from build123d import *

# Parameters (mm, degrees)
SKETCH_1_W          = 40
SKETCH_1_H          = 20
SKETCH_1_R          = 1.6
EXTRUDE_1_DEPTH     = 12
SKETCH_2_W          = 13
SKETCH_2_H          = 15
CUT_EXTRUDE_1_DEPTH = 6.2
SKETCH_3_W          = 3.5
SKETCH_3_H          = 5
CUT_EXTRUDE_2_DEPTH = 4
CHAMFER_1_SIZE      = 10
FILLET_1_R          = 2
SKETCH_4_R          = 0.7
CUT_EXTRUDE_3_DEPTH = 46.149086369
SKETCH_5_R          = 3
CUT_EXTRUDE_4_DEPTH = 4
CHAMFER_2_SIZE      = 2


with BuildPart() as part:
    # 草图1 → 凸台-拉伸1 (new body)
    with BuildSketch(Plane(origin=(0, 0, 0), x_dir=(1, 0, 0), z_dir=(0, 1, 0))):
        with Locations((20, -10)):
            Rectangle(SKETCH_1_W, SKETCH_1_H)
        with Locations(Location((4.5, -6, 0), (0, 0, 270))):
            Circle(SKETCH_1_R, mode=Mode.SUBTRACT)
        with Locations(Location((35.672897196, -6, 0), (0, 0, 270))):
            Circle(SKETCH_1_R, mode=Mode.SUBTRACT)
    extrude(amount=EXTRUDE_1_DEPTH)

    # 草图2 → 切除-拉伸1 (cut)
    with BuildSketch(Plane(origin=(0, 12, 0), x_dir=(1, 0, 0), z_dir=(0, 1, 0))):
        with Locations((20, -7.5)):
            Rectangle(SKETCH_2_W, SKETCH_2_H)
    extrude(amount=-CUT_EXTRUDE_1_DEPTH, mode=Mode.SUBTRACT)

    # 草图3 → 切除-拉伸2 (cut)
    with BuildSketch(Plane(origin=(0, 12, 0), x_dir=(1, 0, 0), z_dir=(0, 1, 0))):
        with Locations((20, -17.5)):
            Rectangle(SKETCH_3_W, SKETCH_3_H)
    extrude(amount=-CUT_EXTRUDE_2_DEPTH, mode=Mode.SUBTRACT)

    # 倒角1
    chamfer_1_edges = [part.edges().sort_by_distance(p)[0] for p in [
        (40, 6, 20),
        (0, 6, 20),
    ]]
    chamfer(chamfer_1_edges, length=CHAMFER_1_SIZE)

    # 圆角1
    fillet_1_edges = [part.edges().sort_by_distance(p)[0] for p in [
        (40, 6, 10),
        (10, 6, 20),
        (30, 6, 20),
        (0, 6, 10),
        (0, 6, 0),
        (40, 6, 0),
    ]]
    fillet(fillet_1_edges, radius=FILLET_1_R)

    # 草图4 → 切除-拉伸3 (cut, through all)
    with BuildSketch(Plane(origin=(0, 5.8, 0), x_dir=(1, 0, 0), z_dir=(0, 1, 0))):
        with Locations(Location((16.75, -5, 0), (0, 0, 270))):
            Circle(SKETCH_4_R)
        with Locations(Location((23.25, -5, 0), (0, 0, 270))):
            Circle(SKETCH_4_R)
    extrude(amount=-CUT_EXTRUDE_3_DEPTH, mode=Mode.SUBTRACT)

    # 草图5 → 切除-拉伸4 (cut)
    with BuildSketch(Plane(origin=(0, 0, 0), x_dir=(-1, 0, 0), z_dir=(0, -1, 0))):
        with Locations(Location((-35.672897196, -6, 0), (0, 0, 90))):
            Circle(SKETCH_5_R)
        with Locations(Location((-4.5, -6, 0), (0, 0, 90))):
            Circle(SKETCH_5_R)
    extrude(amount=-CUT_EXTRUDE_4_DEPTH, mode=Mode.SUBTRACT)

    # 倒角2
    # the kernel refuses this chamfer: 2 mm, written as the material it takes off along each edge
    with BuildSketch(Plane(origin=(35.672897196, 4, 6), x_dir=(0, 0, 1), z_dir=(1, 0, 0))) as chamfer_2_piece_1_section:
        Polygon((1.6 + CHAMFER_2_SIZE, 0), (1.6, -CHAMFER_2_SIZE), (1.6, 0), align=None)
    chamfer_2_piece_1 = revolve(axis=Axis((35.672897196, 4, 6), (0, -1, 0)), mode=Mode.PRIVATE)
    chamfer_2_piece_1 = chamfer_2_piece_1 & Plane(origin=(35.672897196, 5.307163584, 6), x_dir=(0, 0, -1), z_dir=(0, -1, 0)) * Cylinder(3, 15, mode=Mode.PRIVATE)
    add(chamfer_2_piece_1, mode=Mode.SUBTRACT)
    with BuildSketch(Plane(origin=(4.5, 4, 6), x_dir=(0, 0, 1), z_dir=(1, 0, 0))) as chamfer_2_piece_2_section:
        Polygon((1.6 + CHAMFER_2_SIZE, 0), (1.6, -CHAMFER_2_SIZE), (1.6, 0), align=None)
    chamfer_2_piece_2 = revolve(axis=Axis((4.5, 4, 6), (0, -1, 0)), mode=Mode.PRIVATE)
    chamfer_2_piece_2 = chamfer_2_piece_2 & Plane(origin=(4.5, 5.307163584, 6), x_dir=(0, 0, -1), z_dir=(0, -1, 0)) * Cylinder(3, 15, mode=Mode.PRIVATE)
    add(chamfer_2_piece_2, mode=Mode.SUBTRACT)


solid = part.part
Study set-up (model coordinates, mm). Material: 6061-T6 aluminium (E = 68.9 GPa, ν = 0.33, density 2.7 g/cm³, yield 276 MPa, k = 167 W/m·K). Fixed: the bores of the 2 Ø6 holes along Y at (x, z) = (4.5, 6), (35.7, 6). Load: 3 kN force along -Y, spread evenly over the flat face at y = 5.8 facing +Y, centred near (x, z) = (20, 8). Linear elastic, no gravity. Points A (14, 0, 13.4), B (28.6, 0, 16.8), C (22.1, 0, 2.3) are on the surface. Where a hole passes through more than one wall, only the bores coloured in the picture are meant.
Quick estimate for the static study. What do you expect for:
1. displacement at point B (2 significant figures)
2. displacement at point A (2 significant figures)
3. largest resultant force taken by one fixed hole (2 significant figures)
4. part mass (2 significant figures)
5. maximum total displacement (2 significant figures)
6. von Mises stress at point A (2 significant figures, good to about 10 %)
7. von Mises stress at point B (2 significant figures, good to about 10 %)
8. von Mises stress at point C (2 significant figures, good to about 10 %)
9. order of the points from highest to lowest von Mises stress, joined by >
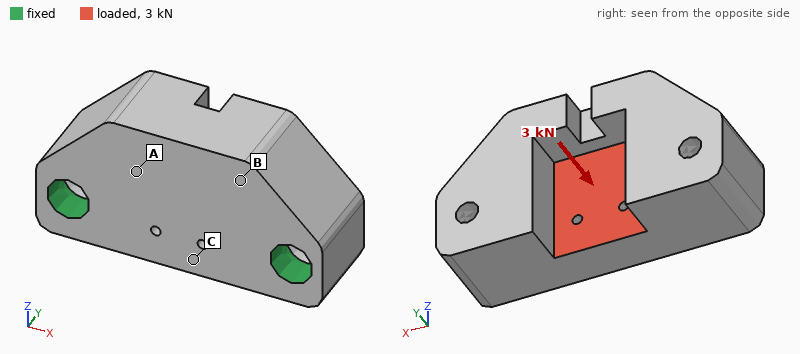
11 µm
13 µm
1.5 kN
18 g
19 µm
20 MPa
10 MPa
54 MPa
C > A > B
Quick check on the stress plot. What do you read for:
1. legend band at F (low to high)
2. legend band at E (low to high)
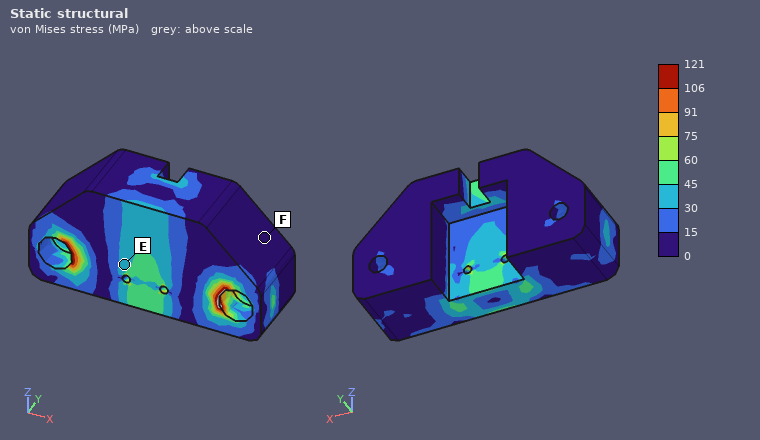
0 to 15 MPa
30 to 45 MPa
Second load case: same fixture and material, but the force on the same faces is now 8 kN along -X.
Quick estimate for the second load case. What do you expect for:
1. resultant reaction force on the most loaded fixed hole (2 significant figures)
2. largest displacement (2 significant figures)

4.1 kN
13 µm
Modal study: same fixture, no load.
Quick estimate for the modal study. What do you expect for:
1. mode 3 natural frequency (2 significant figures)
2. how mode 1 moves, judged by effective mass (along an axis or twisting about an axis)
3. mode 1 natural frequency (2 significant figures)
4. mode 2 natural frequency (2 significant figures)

33 kHz
along Y
19 kHz
31 kHz
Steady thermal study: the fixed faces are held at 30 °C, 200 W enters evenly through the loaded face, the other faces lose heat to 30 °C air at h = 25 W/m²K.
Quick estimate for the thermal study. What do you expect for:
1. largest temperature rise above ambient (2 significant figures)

72 K
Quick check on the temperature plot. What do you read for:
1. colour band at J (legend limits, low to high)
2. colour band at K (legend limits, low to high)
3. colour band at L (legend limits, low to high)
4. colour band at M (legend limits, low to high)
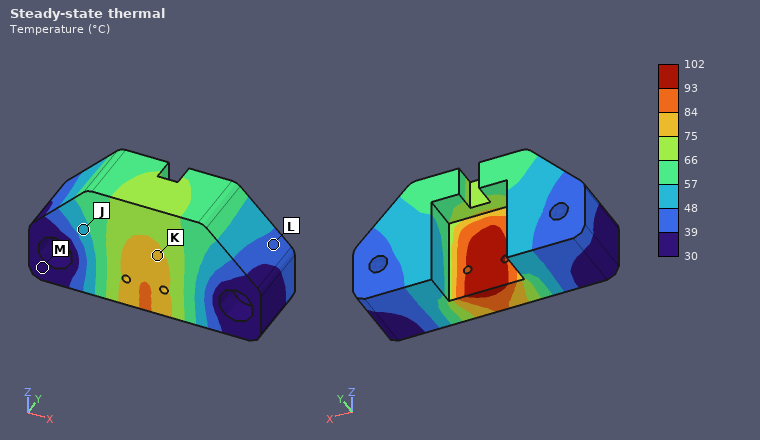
48 to 57 °C
75 to 84 °C
39 to 48 °C
30 to 39 °C
